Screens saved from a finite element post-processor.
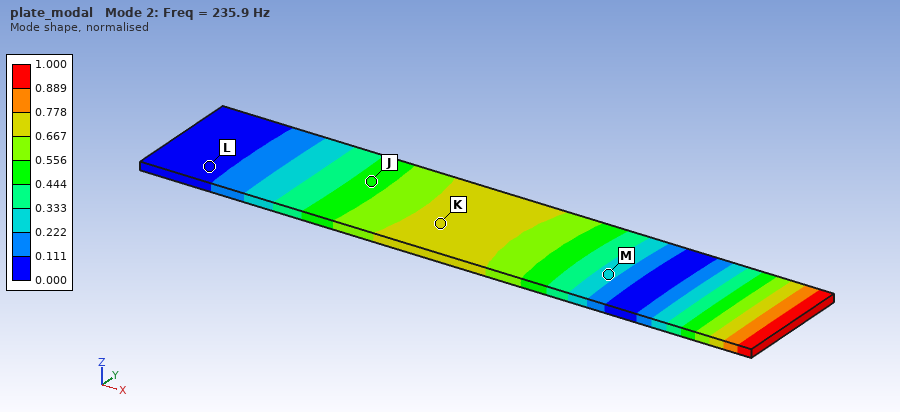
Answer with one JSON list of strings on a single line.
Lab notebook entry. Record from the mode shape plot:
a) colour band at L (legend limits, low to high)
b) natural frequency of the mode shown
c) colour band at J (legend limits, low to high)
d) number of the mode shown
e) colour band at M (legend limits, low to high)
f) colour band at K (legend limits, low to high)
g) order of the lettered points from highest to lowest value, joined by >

["0.000 to 0.111", "235.9 Hz", "0.444 to 0.556", "2", "0.222 to 0.333", "0.667 to 0.778", "K > J > M > L"]
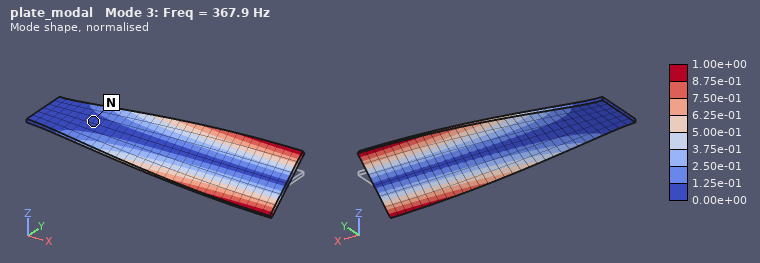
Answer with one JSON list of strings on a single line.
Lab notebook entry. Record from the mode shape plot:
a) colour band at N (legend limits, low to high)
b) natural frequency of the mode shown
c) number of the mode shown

["0.00e+00 to 1.25e-01", "367.9 Hz", "3"]
